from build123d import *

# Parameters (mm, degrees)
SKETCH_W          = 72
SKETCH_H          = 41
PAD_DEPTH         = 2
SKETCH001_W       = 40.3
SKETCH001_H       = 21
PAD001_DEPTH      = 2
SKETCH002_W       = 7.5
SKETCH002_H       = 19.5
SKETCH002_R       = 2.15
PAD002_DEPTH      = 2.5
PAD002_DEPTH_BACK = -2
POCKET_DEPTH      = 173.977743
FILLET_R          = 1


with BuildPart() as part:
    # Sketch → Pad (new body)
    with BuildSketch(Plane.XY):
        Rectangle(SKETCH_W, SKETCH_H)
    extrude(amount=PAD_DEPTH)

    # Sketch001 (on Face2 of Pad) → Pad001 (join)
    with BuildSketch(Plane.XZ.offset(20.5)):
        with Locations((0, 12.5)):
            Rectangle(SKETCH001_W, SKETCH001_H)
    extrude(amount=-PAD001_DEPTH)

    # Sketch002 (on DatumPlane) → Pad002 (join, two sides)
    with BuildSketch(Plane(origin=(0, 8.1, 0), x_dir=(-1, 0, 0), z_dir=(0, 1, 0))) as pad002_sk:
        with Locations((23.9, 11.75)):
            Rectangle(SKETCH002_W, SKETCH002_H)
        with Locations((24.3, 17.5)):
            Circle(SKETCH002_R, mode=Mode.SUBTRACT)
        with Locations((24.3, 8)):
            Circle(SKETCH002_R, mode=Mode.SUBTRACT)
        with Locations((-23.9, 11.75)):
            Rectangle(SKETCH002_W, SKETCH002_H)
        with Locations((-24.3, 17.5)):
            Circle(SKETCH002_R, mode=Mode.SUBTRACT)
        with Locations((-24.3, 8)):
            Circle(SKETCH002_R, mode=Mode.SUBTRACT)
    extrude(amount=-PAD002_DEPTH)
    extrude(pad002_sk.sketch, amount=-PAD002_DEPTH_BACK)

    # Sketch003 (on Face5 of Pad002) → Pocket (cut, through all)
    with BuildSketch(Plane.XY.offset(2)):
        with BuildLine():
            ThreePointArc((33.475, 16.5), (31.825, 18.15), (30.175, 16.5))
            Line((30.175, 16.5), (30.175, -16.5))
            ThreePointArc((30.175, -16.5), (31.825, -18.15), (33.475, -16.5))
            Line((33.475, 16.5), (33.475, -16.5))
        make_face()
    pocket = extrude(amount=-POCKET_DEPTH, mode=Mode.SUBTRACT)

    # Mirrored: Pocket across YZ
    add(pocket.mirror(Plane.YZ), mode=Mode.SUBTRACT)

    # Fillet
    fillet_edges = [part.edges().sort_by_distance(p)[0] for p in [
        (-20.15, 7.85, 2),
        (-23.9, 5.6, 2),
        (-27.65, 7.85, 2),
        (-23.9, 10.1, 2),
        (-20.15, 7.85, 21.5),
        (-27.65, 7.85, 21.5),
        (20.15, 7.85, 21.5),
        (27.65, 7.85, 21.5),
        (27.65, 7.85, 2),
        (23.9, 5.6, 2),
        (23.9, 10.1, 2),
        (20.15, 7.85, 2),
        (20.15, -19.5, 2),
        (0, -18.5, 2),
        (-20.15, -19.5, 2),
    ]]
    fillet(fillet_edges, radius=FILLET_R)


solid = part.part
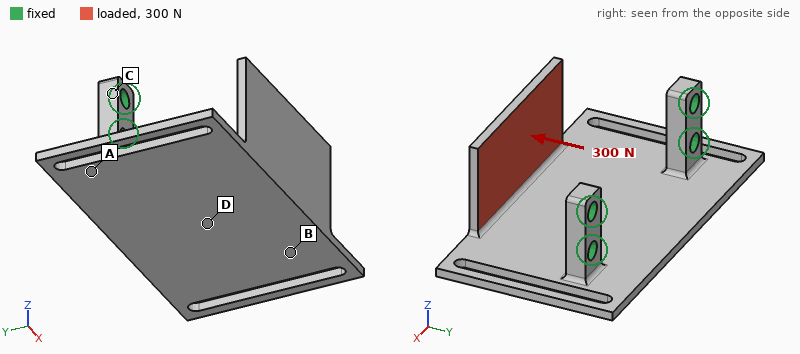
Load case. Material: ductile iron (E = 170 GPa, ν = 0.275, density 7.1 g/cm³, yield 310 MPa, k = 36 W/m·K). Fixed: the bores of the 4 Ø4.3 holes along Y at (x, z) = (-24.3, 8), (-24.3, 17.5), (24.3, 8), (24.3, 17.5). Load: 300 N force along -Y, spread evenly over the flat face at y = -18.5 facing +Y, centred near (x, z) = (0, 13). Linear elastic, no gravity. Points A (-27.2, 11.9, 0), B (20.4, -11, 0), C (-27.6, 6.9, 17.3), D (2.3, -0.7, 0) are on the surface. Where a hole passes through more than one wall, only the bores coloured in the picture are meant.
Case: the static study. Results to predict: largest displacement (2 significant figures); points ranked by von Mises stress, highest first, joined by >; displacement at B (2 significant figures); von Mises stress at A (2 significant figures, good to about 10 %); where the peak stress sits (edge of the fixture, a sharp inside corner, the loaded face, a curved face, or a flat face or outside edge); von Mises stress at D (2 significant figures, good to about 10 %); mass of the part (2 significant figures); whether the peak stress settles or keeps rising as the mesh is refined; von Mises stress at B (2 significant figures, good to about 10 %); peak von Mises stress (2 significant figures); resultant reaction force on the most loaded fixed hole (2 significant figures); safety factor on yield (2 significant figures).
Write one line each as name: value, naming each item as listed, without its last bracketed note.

largest displacement: 0.46 mm
points ranked by von Mises stress, highest first, joined by >: B > D > A > C
displacement at B: 0.11 mm
von Mises stress at A: 25 MPa
where the peak stress sits: a curved face
von Mises stress at D: 59 MPa
mass of the part: 58 g
whether the peak stress settles or keeps rising as the mesh is refined: settles
von Mises stress at B: 73 MPa
peak von Mises stress: 260 MPa
resultant reaction force on the most loaded fixed hole: 150 N
safety factor on yield: 1.2
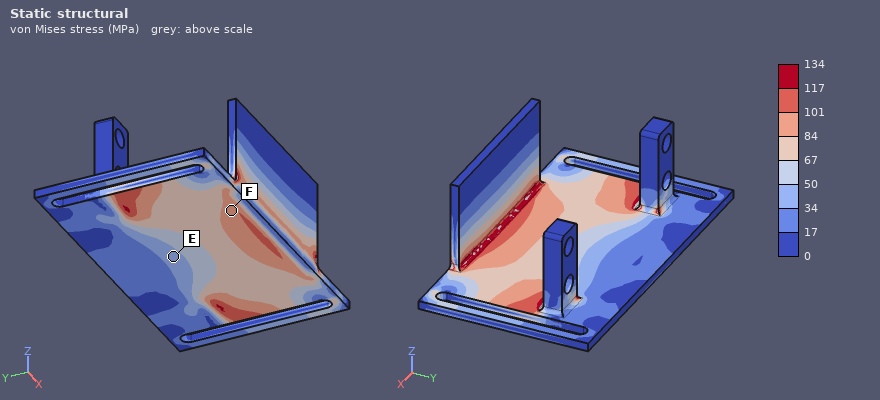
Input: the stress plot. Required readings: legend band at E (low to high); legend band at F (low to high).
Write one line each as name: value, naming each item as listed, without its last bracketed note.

legend band at E: 34 to 50 MPa
legend band at F: 84 to 101 MPa
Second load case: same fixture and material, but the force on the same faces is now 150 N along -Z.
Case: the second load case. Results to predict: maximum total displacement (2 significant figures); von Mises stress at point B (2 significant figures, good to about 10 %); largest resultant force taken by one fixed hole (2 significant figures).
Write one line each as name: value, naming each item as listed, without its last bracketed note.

maximum total displacement: 0.26 mm
von Mises stress at point B: 29 MPa
largest resultant force taken by one fixed hole: 83 N
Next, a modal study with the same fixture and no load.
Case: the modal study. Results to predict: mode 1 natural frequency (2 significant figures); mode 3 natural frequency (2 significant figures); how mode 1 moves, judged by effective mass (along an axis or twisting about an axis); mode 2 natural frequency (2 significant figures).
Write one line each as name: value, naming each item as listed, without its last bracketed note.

mode 1 natural frequency: 900 Hz
mode 3 natural frequency: 2500 Hz
how mode 1 moves, judged by effective mass: along Z
mode 2 natural frequency: 1800 Hz
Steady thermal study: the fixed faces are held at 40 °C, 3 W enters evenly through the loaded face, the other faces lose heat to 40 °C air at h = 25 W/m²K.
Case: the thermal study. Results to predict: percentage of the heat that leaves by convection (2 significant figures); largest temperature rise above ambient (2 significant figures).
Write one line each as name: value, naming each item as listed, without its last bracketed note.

percentage of the heat that leaves by convection: 57 %
largest temperature rise above ambient: 26 K
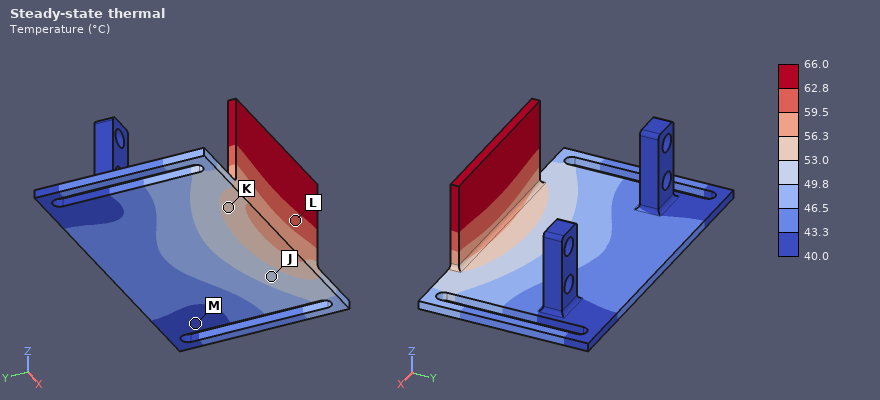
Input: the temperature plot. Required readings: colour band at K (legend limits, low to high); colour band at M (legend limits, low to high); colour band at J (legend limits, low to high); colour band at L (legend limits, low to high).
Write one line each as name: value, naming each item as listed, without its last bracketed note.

colour band at K: 53.0 to 56.3 °C
colour band at M: 40.0 to 43.3 °C
colour band at J: 49.8 to 53.0 °C
colour band at L: 59.5 to 62.8 °C
